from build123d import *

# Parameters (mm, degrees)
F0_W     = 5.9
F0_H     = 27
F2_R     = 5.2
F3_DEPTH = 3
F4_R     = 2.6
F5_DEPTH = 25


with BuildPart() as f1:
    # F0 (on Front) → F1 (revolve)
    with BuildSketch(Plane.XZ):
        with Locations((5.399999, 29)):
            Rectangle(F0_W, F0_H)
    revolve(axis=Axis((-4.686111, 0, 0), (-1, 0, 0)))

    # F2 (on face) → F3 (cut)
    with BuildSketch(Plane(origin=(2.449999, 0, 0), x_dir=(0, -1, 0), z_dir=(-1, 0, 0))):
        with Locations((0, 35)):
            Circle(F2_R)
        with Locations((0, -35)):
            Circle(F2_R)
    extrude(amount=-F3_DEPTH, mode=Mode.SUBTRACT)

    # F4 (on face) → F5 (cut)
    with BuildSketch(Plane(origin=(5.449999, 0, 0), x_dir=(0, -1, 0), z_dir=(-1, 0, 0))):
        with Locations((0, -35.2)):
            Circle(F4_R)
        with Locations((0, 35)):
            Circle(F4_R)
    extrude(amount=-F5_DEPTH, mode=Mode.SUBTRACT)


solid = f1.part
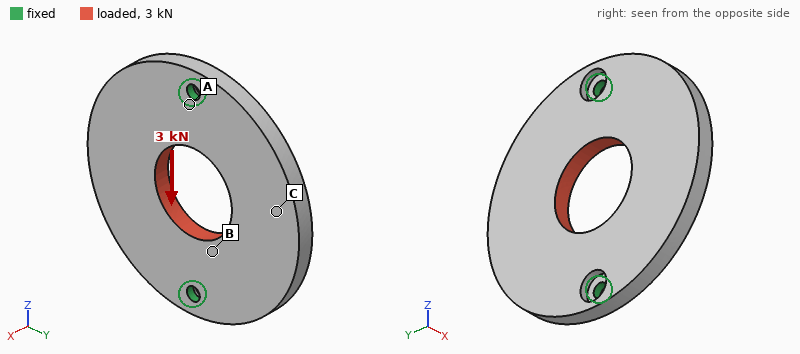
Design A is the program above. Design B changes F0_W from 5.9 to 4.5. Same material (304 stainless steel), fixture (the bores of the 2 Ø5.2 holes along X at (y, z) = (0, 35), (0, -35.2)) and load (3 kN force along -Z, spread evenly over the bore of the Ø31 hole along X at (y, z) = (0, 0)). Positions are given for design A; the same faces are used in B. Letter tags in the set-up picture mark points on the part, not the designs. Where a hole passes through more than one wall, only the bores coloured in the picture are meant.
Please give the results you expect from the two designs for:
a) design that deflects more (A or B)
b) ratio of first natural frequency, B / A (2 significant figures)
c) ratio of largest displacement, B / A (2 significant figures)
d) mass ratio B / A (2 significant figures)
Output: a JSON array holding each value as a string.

["B", "0.82", "1.3", "0.76"]
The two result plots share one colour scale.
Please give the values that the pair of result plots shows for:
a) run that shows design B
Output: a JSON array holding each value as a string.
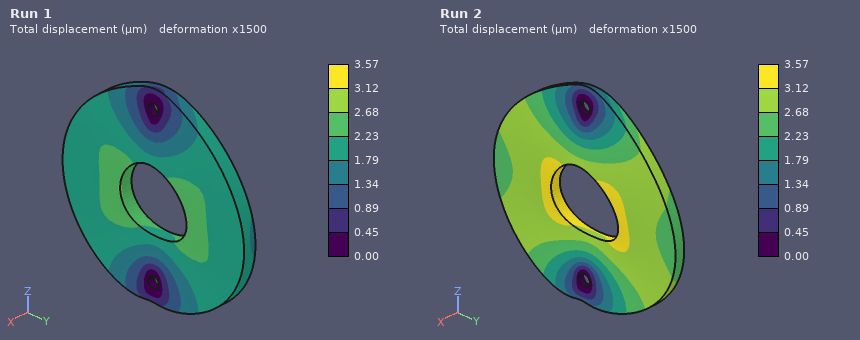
["Run 2"]
